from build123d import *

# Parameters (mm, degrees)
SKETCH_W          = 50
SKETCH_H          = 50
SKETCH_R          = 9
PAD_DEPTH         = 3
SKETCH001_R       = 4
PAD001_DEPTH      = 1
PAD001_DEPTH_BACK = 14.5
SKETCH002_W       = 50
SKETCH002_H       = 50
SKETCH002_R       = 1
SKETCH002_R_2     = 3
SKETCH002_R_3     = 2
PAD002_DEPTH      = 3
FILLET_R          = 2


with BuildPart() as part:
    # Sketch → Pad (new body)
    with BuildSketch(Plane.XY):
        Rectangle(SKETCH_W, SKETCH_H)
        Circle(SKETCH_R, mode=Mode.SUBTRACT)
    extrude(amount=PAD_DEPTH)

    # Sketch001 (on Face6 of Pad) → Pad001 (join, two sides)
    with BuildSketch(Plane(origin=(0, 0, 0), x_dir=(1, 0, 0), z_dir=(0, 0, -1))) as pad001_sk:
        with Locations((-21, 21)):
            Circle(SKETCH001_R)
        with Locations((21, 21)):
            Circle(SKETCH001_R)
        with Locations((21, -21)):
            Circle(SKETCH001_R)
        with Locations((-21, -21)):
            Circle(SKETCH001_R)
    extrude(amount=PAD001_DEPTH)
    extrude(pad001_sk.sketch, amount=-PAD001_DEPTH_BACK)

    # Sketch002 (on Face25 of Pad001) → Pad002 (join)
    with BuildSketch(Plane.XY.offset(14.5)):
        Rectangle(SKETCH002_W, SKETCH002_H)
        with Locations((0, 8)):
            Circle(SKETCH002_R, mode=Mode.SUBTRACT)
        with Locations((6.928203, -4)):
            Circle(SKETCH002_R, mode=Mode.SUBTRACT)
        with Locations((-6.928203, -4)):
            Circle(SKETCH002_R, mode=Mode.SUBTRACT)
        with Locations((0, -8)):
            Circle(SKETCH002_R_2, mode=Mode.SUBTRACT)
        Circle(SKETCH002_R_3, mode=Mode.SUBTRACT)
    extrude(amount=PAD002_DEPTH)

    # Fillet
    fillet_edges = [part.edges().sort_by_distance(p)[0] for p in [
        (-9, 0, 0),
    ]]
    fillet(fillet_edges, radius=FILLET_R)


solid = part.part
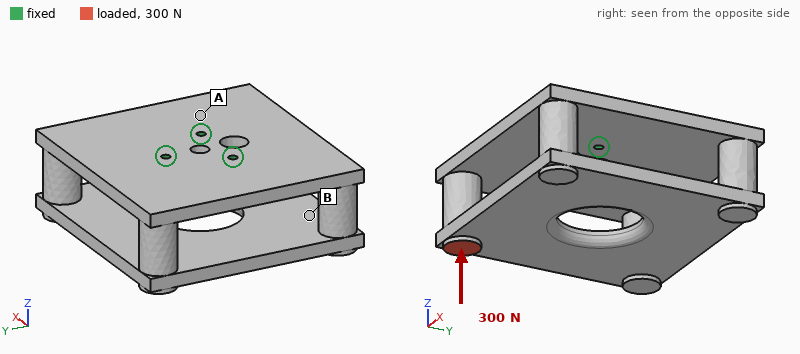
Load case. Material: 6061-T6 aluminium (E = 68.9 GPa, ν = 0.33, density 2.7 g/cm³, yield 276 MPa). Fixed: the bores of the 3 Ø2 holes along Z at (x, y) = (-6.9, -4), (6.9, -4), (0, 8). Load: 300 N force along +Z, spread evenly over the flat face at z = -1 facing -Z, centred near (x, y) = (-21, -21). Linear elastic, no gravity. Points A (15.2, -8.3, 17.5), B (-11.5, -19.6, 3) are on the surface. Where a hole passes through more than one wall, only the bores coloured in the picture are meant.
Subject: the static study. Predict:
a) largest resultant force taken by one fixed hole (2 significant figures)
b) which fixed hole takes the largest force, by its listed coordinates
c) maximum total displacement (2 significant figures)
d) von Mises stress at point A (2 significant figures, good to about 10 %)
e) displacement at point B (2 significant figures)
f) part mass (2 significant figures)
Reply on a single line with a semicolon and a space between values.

540 N; (-6.9, -4); 0.17 mm; 18 MPa; 0.12 mm; 45 g
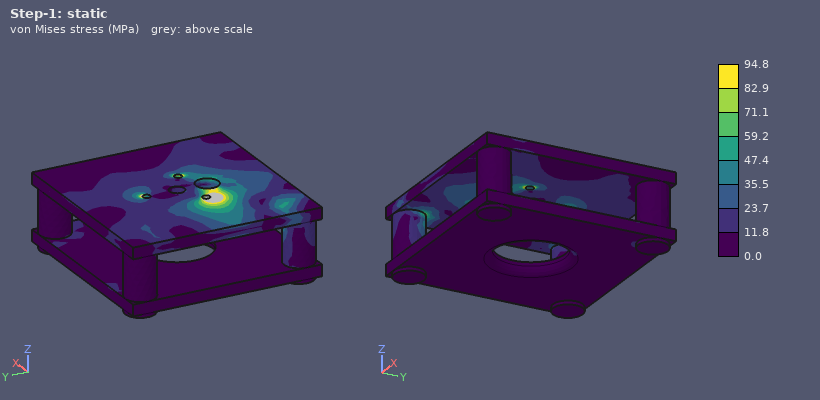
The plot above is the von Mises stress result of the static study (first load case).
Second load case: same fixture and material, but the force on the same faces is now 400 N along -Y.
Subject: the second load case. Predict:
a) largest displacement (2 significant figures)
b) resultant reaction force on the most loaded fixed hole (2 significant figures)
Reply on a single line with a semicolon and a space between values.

0.15 mm; 490 N
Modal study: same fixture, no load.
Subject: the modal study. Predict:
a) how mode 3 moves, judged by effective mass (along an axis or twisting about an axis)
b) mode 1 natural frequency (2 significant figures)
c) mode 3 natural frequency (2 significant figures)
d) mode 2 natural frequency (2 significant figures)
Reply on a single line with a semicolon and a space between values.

along Z; 1900 Hz; 2900 Hz; 1900 Hz
